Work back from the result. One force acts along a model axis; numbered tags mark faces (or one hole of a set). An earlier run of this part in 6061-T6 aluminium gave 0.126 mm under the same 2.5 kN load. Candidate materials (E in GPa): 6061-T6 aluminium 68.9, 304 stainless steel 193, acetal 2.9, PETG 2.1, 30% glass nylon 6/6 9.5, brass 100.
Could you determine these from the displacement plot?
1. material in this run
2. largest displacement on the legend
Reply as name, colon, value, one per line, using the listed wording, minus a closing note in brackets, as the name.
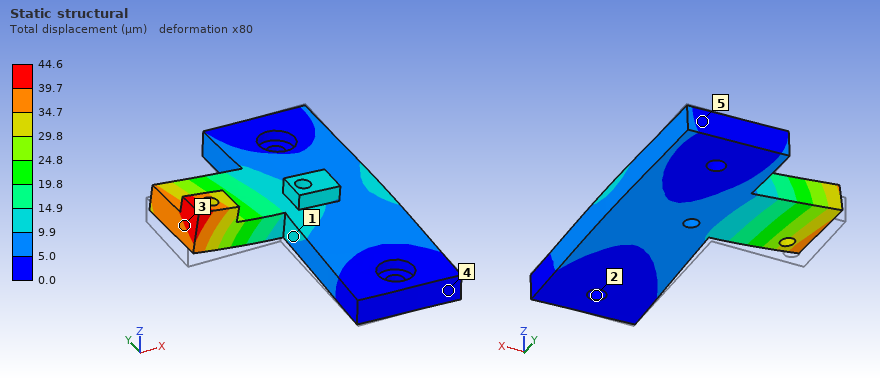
material in this run: 304 stainless steel
largest displacement on the legend: 44.6 µm
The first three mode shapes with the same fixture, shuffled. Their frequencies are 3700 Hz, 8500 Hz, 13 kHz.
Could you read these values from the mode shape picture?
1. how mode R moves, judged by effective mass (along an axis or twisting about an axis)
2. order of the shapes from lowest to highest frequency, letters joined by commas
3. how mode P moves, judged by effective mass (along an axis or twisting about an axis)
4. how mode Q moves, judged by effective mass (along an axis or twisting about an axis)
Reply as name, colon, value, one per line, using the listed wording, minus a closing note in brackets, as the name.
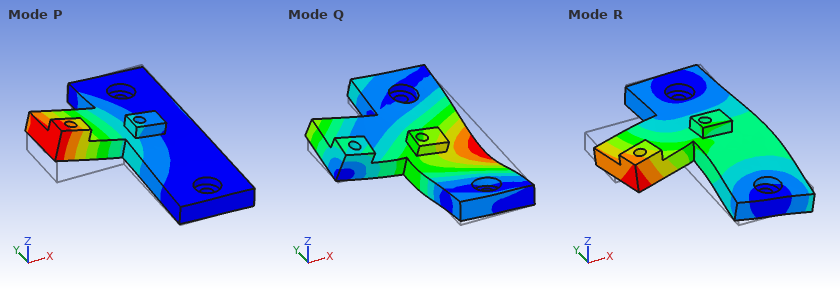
how mode R moves, judged by effective mass: along X
order of the shapes from lowest to highest frequency, letters joined by commas: P, Q, R
how mode P moves, judged by effective mass: along Z
how mode Q moves, judged by effective mass: along Z
